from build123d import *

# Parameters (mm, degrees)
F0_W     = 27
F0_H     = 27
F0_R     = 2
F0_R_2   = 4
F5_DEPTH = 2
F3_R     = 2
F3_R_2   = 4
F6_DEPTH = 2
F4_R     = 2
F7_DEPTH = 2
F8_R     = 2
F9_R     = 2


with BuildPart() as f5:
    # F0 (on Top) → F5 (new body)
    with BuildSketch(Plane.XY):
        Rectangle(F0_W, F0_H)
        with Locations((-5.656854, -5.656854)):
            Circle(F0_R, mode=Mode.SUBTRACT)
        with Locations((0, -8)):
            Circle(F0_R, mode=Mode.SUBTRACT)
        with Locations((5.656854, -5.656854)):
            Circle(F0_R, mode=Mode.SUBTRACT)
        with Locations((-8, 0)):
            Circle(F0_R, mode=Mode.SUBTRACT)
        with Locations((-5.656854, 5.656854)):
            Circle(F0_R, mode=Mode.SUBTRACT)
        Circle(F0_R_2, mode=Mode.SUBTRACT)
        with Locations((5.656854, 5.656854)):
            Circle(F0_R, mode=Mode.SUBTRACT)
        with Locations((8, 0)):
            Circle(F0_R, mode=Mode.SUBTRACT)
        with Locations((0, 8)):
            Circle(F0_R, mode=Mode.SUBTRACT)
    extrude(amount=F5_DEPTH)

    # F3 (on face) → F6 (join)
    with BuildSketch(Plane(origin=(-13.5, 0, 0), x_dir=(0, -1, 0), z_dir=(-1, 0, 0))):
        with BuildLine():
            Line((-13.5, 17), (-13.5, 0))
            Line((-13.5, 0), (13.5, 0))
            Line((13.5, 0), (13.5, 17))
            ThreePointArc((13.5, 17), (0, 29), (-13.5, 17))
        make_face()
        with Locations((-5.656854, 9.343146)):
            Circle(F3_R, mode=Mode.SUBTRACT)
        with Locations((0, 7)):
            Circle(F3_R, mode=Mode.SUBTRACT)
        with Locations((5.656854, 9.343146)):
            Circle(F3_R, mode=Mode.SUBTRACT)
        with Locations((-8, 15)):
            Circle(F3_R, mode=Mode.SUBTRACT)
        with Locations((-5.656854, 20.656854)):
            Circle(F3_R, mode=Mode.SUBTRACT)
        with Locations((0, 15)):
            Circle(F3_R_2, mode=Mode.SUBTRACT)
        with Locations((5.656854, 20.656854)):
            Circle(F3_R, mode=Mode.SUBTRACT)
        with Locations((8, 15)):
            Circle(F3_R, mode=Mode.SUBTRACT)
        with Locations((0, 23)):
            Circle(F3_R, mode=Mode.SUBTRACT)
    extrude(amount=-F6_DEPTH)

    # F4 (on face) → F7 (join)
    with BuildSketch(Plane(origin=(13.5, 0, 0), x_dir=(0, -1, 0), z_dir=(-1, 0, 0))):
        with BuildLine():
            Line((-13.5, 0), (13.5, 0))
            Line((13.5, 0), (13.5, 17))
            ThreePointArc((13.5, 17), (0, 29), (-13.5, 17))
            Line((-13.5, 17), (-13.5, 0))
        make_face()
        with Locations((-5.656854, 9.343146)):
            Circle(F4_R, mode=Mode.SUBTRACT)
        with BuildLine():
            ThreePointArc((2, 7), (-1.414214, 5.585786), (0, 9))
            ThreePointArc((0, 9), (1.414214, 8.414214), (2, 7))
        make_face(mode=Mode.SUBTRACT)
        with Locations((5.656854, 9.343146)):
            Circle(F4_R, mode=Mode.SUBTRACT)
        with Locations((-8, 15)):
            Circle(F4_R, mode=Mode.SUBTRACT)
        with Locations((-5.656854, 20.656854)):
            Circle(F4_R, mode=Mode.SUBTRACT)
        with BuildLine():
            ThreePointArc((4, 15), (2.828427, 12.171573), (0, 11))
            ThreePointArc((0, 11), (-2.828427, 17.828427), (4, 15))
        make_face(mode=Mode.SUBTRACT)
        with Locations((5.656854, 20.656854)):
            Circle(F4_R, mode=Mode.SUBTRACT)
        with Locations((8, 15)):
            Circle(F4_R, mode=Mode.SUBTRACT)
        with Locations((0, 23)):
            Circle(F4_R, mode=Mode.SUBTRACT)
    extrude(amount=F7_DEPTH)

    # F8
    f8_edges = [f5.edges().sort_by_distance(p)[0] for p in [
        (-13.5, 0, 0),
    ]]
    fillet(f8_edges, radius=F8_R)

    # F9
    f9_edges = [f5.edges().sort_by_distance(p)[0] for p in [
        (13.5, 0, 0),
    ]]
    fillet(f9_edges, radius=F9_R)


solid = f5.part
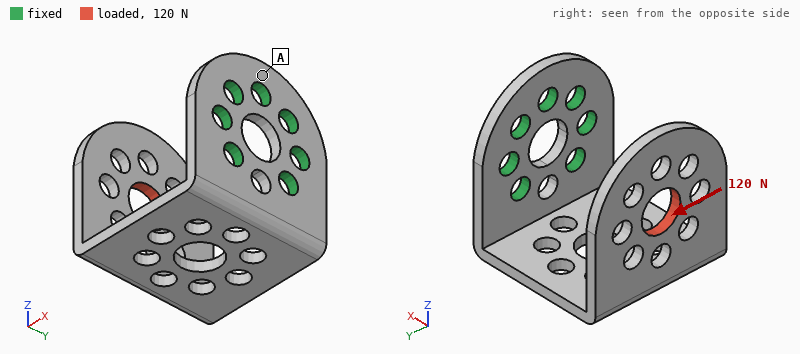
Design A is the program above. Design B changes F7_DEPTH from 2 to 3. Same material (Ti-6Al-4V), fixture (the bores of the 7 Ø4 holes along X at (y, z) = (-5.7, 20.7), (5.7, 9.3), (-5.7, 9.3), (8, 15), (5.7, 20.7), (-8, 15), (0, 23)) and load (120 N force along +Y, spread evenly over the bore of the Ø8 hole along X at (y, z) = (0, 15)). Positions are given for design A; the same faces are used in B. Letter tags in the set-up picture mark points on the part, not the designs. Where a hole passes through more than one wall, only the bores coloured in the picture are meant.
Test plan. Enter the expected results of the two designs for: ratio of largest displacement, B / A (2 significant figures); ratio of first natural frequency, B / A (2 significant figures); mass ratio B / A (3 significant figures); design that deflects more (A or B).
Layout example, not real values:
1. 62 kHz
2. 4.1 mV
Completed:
1. 0.75
2. 1.1
3. 1.16
4. A
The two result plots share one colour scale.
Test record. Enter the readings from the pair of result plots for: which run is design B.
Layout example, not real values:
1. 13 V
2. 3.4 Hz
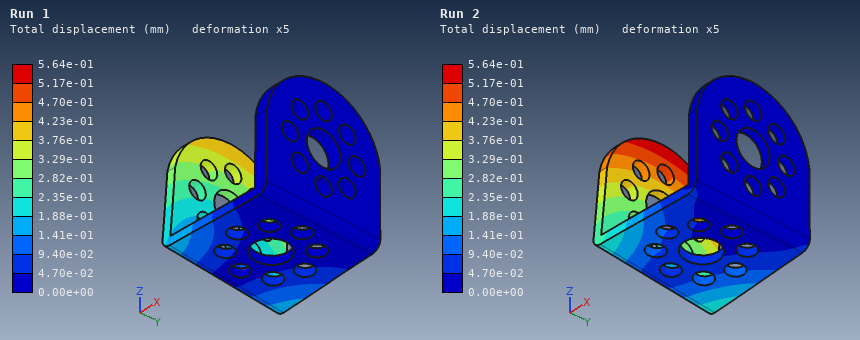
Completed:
1. Run 1
